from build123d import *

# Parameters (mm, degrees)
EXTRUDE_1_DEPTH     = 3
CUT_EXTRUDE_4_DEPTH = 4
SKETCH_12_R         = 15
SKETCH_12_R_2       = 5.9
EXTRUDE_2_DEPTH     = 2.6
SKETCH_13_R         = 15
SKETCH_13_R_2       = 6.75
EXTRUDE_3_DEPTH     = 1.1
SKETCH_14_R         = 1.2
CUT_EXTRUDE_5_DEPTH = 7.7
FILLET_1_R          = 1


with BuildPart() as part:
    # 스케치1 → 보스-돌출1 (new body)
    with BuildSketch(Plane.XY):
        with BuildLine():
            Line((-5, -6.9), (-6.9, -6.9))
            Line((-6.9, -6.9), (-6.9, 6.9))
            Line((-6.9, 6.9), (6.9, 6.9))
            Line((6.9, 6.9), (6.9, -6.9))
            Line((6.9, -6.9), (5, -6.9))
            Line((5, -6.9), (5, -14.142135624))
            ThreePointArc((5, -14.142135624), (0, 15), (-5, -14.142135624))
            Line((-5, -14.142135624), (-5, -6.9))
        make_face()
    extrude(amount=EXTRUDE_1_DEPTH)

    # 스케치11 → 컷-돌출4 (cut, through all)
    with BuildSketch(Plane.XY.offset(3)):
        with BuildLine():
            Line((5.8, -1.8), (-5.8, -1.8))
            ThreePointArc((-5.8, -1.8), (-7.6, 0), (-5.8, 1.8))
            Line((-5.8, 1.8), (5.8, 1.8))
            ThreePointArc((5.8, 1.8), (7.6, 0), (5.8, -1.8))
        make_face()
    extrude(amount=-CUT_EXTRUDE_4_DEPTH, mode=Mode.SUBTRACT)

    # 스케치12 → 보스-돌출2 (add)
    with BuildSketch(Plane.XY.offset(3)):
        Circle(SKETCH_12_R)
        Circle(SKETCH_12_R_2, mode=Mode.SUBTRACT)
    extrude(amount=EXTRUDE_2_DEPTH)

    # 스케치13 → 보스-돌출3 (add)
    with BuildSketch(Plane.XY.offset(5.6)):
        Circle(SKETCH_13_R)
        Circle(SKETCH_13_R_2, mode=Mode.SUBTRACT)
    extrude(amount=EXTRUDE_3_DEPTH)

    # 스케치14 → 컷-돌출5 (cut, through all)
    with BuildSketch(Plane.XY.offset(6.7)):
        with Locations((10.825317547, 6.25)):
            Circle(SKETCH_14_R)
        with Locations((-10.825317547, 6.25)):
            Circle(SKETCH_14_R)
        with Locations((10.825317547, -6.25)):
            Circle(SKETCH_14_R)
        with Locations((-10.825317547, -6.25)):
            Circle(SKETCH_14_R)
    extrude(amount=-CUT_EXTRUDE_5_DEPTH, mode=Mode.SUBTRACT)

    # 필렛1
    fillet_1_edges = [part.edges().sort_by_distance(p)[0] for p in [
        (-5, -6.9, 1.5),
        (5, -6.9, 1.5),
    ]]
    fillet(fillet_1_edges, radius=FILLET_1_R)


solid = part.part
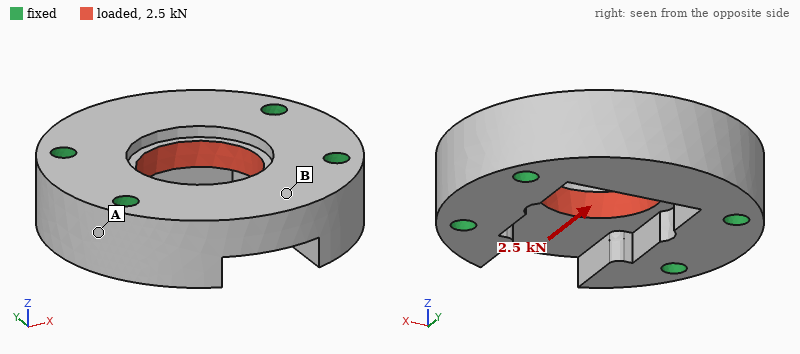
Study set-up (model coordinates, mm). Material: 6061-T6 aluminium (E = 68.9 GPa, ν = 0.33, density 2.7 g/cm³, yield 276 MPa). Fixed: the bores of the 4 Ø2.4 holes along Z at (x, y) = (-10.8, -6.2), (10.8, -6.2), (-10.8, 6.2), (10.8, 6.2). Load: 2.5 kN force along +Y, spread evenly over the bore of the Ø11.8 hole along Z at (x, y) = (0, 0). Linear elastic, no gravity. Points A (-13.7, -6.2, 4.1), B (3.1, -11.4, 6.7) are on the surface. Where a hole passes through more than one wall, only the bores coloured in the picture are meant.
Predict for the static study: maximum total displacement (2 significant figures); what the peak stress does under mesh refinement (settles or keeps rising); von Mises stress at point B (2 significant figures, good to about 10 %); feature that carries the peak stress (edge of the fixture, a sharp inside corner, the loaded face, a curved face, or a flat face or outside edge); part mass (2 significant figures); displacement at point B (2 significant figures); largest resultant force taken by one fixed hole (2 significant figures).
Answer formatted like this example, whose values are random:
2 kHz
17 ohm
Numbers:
5.9 µm
keeps rising
13 MPa
edge of the fixture
9.1 g
3.9 µm
640 N
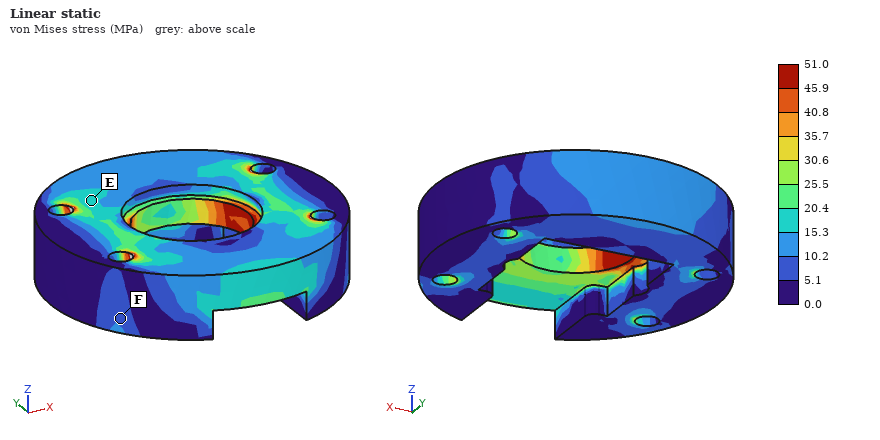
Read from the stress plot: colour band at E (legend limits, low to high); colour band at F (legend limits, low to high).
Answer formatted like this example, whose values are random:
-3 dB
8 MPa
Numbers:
15.3 to 20.4 MPa
5.1 to 10.2 MPa
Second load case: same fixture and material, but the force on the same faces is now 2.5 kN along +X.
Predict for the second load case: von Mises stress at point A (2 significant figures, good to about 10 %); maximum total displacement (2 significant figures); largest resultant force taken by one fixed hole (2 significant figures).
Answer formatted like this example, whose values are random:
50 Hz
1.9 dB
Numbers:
6.5 MPa
3.1 µm
640 N
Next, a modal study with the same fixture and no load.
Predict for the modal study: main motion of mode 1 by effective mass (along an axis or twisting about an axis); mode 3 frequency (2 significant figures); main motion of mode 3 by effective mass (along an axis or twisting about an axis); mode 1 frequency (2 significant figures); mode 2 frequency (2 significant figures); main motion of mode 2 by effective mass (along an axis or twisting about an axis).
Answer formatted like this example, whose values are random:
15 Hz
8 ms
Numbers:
along Z
61 kHz
along Y
36 kHz
40 kHz
along Z
